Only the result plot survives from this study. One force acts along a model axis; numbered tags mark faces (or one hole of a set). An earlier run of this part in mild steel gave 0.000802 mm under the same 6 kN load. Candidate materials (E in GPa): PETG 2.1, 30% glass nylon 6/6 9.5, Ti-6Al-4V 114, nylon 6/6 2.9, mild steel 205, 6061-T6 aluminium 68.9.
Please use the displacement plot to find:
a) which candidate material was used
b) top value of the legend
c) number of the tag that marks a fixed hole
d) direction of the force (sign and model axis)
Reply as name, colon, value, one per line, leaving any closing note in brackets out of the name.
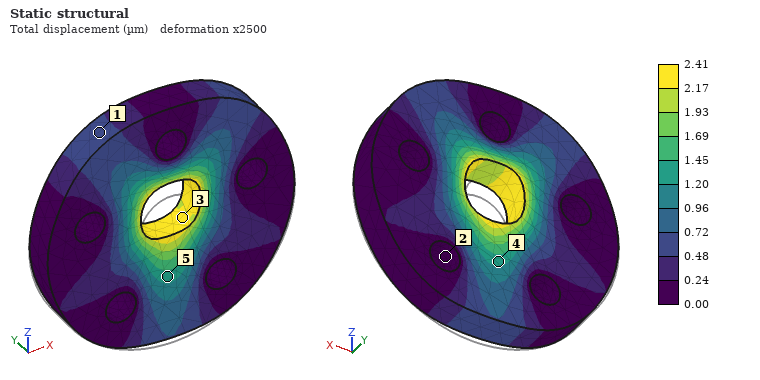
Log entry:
which candidate material was used: 6061-T6 aluminium
top value of the legend: 2.41 µm
number of the tag that marks a fixed hole: 2
direction of the force: +Z
